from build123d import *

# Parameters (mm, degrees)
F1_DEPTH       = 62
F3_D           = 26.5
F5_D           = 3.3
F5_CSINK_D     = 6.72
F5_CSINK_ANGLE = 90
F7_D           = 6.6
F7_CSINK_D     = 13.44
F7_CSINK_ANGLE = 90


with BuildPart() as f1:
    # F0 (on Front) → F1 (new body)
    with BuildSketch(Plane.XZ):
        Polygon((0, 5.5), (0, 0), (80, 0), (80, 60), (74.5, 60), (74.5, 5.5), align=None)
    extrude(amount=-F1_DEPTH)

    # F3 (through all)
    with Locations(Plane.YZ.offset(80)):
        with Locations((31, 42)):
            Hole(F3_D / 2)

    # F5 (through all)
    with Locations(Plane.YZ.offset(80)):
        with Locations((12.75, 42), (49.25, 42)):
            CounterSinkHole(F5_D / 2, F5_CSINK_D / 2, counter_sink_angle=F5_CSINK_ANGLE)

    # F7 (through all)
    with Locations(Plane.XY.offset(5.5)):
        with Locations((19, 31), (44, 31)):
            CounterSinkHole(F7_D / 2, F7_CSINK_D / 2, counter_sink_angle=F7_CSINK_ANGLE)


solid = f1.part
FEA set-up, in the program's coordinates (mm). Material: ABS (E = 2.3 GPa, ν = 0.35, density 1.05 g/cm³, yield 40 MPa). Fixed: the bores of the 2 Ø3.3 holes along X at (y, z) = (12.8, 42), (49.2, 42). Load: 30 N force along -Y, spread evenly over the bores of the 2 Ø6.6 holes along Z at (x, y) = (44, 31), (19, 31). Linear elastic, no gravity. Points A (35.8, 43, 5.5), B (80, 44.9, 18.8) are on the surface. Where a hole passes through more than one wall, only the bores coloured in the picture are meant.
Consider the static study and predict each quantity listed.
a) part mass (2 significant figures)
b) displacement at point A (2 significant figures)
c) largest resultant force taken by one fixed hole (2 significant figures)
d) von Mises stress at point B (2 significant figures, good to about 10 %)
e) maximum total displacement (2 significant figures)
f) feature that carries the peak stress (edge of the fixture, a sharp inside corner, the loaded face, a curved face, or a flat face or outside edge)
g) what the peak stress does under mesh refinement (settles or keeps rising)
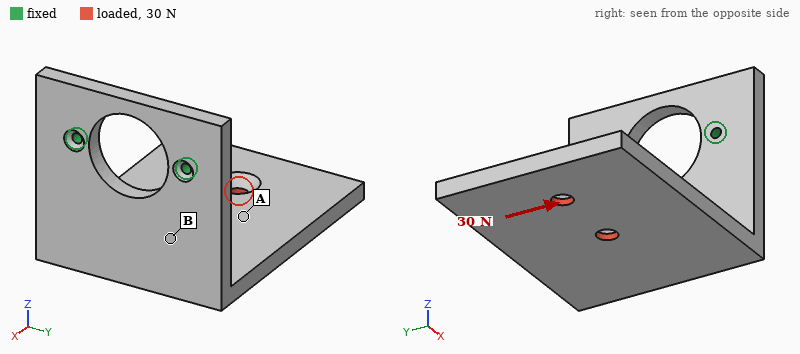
44 g
0.56 mm
44 N
2.6 MPa
1.1 mm
edge of the fixture
keeps rising
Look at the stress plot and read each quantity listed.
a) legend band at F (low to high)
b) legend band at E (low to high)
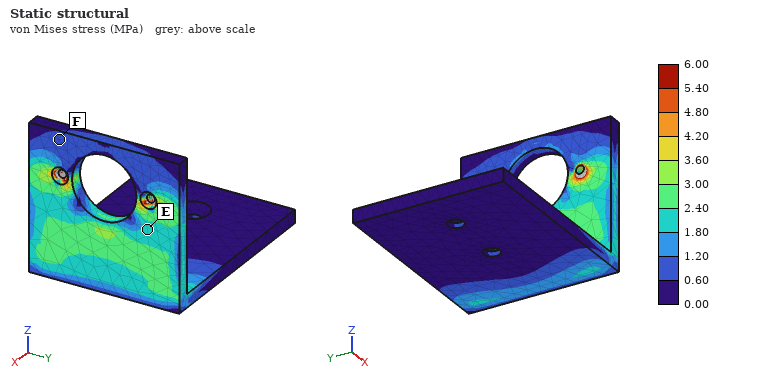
0.60 to 1.20 MPa
1.80 to 2.40 MPa
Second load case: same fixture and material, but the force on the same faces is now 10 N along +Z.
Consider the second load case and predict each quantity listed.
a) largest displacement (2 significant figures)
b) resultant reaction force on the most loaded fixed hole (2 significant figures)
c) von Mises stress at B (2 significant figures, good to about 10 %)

1.3 mm
5.3 N
1.3 MPa
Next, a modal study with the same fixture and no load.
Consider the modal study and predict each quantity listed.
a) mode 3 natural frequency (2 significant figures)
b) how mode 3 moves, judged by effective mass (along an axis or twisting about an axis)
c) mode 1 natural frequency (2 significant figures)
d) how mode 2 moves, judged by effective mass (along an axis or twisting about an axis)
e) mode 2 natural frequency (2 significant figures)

350 Hz
along X
100 Hz
along Y
210 Hz
